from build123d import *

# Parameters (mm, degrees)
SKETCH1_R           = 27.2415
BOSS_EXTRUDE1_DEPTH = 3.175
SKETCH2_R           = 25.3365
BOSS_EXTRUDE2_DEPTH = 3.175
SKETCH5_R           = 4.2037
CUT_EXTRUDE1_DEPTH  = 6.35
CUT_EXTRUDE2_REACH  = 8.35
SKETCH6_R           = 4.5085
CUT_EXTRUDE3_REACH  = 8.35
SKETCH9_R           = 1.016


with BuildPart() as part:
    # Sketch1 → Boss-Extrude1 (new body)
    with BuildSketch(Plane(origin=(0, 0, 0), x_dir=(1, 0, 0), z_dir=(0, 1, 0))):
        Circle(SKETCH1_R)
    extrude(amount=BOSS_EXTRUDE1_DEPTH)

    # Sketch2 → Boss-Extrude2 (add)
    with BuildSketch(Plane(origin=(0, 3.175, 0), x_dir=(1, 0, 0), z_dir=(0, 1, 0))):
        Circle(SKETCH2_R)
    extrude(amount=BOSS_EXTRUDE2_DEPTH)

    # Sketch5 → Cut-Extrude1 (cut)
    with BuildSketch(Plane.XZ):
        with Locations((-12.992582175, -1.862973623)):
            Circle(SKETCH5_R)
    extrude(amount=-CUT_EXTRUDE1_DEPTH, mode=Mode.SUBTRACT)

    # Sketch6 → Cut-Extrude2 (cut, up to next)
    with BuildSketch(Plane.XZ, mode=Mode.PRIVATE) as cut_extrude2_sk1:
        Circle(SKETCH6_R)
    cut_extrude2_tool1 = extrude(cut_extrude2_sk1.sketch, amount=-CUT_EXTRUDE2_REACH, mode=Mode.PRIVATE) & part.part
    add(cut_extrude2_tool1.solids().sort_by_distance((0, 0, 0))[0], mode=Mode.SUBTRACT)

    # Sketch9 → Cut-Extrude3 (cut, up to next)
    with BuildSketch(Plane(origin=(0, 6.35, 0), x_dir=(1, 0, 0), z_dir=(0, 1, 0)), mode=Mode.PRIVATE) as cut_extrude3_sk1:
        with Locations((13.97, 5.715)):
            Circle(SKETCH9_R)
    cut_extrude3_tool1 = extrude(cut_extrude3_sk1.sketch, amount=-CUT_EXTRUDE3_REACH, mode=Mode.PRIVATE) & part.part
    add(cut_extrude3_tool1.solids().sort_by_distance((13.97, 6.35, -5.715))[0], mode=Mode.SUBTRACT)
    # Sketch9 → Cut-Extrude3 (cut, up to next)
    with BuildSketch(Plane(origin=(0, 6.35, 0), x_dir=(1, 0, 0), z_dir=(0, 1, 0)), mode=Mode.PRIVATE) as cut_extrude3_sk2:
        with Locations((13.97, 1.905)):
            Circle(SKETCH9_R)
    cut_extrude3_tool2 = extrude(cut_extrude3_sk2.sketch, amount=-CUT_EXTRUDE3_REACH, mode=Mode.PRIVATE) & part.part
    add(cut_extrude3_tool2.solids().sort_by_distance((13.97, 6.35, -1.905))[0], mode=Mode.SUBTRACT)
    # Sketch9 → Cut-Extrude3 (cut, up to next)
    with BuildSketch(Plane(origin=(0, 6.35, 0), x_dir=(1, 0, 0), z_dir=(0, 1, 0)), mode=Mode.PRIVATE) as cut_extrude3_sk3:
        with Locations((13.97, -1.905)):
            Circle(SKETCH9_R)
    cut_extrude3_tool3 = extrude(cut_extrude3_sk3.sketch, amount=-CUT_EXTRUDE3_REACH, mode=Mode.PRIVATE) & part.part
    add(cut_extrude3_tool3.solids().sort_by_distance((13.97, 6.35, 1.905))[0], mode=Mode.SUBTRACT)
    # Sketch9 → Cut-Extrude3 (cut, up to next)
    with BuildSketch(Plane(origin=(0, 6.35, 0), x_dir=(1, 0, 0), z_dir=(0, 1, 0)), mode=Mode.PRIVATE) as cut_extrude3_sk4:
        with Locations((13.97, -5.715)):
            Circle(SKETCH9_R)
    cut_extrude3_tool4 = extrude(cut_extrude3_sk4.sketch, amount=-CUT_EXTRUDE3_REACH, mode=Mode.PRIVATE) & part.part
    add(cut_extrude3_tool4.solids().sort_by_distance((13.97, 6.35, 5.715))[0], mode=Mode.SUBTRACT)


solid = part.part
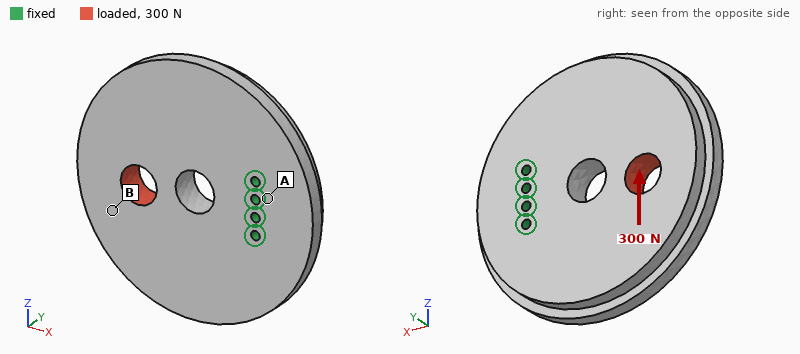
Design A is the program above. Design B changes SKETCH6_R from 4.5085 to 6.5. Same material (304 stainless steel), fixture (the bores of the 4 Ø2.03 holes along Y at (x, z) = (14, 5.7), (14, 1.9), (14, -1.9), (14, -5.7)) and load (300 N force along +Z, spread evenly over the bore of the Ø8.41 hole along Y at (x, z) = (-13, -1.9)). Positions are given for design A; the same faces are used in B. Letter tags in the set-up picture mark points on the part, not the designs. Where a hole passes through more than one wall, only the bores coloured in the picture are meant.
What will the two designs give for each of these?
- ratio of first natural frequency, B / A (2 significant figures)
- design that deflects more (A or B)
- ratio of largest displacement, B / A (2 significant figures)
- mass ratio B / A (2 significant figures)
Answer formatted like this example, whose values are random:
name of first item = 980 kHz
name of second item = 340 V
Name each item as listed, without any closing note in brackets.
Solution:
ratio of first natural frequency, B / A = 0.94
design that deflects more = B
ratio of largest displacement, B / A = 1.2
mass ratio B / A = 0.97
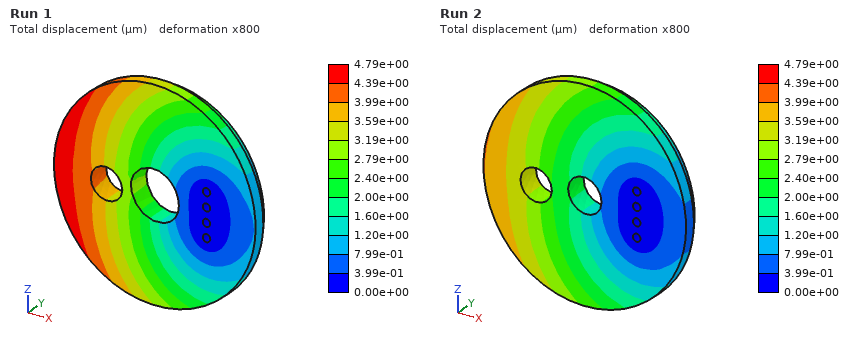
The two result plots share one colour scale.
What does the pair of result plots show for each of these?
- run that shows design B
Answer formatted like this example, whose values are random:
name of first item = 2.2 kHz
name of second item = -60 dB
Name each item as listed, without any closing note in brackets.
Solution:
run that shows design B = Run 1
